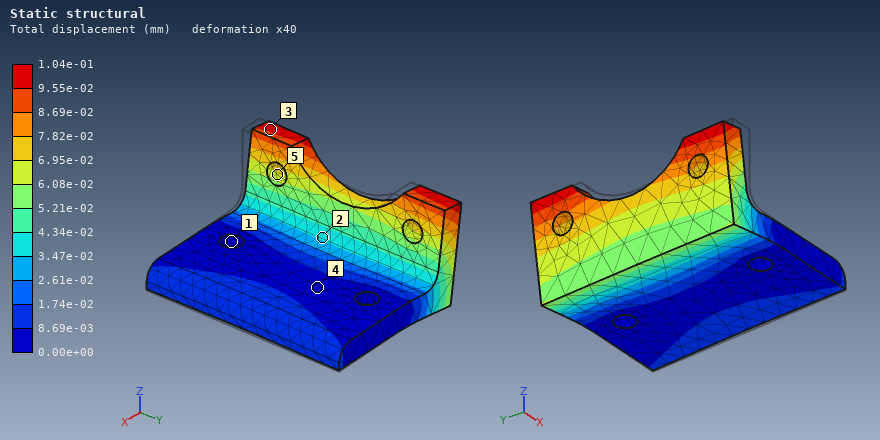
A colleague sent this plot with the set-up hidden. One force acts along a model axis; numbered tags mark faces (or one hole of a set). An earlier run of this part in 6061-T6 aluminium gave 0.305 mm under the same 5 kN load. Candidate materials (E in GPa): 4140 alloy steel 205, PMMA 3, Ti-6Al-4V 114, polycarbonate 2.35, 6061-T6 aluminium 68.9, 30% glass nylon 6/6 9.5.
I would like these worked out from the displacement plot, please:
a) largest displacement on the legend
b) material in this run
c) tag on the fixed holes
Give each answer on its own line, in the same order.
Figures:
1.04e-01 mm
4140 alloy steel
1
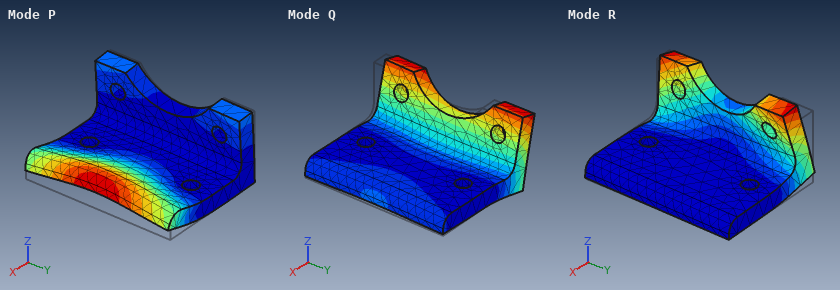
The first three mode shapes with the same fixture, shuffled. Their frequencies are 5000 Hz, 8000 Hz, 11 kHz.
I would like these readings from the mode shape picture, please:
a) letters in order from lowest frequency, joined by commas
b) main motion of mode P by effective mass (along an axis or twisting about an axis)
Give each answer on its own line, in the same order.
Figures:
Q, R, P
along Z
